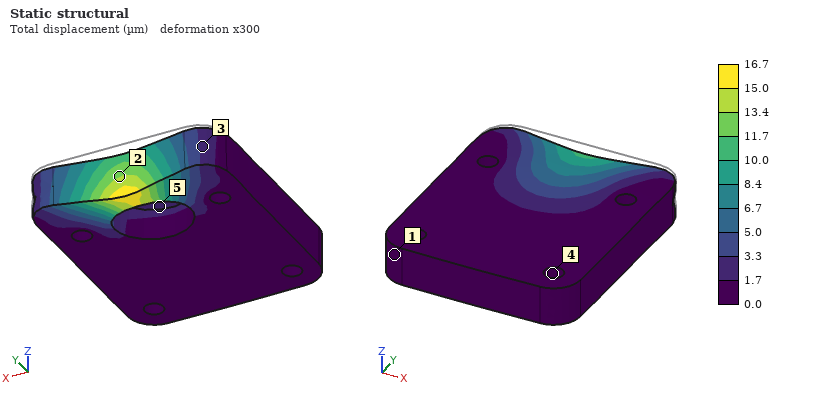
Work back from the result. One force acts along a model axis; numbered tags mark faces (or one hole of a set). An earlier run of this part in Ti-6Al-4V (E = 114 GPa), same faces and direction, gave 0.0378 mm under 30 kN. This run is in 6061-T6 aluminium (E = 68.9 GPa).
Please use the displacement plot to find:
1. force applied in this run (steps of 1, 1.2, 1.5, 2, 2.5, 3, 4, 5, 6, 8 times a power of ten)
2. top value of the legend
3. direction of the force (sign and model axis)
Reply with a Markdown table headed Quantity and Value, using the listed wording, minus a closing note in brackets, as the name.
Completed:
| Quantity | Value |
|---|---|
| force applied in this run | 8 kN |
| top value of the legend | 16.7 µm |
| direction of the force | -Y |
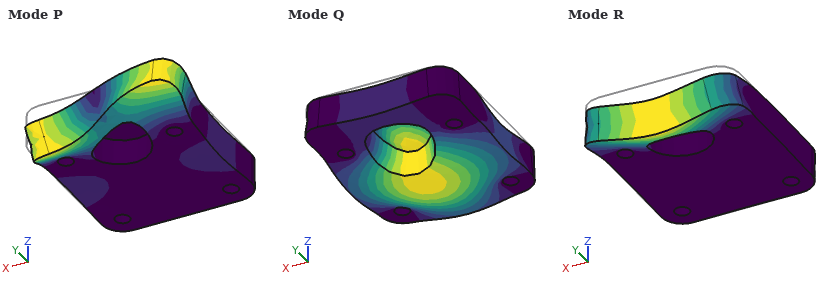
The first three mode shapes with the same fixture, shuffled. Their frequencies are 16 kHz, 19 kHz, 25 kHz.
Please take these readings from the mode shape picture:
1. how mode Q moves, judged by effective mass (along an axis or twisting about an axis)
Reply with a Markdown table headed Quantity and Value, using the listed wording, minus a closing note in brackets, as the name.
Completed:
| Quantity | Value |
|---|---|
| how mode Q moves, judged by effective mass | along Z |
